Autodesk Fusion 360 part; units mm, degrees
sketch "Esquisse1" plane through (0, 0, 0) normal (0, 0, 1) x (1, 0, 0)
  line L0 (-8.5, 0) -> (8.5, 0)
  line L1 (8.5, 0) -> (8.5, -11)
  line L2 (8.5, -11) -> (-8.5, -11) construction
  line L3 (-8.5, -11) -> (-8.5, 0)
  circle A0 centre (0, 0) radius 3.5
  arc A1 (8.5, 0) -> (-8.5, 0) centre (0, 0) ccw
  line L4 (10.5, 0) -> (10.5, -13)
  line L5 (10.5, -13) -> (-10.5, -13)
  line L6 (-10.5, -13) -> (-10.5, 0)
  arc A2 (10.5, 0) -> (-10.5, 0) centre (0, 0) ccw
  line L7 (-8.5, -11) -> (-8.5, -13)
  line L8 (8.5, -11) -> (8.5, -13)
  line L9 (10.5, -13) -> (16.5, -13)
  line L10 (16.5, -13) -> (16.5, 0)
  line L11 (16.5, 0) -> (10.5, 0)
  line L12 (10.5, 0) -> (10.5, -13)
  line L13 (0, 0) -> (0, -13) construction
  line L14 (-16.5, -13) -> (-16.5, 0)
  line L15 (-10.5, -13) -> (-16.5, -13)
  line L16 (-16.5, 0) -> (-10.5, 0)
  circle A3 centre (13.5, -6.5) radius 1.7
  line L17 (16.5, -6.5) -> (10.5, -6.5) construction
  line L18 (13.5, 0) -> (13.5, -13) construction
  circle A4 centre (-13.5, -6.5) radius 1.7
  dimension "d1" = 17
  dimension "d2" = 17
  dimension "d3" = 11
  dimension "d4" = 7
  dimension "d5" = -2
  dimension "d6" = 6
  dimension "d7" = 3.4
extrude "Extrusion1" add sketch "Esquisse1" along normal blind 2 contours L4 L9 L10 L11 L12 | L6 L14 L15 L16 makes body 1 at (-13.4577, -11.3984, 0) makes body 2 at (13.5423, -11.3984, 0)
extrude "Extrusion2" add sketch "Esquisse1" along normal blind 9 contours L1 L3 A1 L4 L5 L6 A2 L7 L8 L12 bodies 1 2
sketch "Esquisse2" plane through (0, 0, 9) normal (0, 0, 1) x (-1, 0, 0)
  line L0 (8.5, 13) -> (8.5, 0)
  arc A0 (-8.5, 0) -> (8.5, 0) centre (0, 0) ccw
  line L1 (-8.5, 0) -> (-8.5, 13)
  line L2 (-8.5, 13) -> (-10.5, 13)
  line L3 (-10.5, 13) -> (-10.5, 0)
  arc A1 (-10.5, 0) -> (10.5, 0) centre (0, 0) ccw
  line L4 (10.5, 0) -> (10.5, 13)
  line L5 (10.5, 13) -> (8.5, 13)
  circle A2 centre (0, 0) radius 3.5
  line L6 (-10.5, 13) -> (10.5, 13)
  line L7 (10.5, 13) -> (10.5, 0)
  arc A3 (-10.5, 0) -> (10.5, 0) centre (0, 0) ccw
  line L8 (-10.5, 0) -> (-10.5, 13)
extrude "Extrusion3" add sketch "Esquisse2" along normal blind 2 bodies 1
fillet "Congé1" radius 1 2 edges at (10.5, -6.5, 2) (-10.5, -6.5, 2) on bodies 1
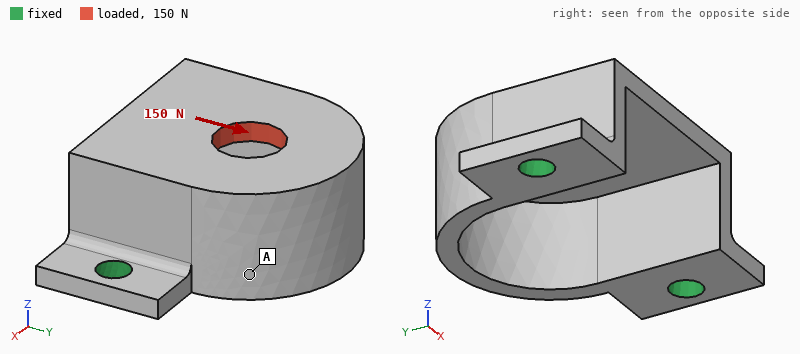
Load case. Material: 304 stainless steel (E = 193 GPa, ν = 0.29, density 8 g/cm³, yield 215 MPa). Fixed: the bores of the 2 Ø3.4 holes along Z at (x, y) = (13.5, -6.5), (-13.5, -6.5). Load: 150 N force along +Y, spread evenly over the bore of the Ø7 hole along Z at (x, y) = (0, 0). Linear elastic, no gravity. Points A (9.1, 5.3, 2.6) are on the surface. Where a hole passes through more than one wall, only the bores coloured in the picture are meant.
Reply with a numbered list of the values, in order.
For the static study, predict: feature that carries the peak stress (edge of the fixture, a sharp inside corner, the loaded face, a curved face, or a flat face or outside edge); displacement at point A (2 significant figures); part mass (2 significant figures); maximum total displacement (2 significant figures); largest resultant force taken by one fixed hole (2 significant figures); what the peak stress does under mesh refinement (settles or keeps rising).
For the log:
1. edge of the fixture
2. 6.9 µm
3. 17 g
4. 12 µm
5. 75 N
6. keeps rising
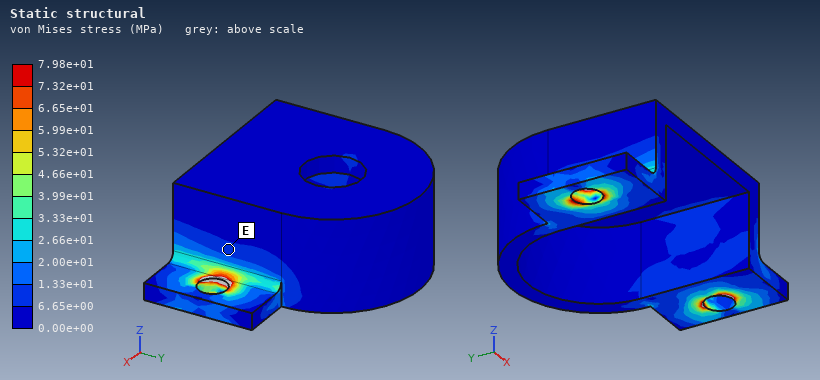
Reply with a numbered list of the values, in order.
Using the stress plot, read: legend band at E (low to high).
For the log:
1. 6.65e+00 to 1.33e+01 MPa
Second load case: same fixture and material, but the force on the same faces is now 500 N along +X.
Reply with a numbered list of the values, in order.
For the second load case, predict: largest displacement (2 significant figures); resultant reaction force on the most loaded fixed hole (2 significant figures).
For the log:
1. 14 µm
2. 310 N
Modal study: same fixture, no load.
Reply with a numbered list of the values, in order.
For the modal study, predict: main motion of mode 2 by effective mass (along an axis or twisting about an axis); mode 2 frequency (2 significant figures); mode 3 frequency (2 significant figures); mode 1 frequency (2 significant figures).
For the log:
1. along X
2. 11 kHz
3. 14 kHz
4. 5500 Hz
